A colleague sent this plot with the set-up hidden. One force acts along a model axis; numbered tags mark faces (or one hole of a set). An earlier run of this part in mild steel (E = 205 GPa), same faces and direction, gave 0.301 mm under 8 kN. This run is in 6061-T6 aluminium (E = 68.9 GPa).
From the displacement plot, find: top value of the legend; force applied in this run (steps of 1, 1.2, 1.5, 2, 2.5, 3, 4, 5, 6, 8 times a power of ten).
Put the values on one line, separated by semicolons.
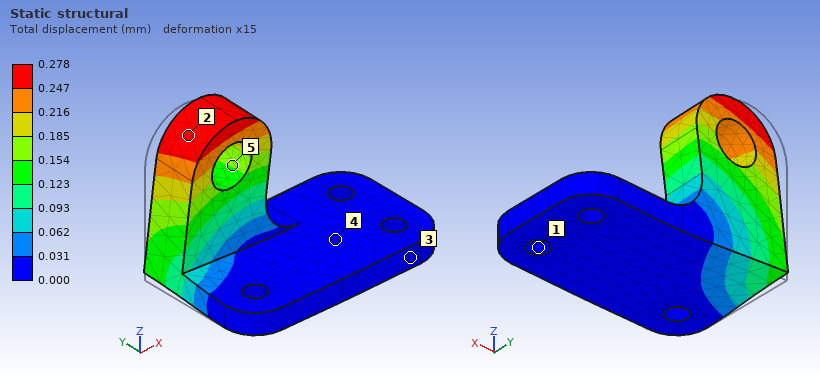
0.278 mm; 2.5 kN
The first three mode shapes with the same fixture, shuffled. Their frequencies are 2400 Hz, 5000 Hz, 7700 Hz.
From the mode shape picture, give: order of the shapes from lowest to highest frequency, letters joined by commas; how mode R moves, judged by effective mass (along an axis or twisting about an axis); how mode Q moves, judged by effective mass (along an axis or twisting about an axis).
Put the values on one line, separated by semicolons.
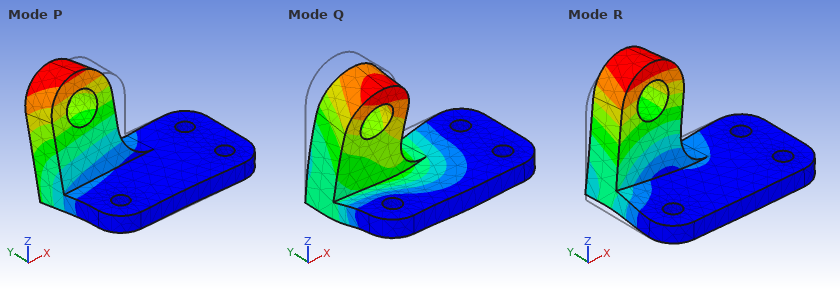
P, R, Q; along X; along Z
